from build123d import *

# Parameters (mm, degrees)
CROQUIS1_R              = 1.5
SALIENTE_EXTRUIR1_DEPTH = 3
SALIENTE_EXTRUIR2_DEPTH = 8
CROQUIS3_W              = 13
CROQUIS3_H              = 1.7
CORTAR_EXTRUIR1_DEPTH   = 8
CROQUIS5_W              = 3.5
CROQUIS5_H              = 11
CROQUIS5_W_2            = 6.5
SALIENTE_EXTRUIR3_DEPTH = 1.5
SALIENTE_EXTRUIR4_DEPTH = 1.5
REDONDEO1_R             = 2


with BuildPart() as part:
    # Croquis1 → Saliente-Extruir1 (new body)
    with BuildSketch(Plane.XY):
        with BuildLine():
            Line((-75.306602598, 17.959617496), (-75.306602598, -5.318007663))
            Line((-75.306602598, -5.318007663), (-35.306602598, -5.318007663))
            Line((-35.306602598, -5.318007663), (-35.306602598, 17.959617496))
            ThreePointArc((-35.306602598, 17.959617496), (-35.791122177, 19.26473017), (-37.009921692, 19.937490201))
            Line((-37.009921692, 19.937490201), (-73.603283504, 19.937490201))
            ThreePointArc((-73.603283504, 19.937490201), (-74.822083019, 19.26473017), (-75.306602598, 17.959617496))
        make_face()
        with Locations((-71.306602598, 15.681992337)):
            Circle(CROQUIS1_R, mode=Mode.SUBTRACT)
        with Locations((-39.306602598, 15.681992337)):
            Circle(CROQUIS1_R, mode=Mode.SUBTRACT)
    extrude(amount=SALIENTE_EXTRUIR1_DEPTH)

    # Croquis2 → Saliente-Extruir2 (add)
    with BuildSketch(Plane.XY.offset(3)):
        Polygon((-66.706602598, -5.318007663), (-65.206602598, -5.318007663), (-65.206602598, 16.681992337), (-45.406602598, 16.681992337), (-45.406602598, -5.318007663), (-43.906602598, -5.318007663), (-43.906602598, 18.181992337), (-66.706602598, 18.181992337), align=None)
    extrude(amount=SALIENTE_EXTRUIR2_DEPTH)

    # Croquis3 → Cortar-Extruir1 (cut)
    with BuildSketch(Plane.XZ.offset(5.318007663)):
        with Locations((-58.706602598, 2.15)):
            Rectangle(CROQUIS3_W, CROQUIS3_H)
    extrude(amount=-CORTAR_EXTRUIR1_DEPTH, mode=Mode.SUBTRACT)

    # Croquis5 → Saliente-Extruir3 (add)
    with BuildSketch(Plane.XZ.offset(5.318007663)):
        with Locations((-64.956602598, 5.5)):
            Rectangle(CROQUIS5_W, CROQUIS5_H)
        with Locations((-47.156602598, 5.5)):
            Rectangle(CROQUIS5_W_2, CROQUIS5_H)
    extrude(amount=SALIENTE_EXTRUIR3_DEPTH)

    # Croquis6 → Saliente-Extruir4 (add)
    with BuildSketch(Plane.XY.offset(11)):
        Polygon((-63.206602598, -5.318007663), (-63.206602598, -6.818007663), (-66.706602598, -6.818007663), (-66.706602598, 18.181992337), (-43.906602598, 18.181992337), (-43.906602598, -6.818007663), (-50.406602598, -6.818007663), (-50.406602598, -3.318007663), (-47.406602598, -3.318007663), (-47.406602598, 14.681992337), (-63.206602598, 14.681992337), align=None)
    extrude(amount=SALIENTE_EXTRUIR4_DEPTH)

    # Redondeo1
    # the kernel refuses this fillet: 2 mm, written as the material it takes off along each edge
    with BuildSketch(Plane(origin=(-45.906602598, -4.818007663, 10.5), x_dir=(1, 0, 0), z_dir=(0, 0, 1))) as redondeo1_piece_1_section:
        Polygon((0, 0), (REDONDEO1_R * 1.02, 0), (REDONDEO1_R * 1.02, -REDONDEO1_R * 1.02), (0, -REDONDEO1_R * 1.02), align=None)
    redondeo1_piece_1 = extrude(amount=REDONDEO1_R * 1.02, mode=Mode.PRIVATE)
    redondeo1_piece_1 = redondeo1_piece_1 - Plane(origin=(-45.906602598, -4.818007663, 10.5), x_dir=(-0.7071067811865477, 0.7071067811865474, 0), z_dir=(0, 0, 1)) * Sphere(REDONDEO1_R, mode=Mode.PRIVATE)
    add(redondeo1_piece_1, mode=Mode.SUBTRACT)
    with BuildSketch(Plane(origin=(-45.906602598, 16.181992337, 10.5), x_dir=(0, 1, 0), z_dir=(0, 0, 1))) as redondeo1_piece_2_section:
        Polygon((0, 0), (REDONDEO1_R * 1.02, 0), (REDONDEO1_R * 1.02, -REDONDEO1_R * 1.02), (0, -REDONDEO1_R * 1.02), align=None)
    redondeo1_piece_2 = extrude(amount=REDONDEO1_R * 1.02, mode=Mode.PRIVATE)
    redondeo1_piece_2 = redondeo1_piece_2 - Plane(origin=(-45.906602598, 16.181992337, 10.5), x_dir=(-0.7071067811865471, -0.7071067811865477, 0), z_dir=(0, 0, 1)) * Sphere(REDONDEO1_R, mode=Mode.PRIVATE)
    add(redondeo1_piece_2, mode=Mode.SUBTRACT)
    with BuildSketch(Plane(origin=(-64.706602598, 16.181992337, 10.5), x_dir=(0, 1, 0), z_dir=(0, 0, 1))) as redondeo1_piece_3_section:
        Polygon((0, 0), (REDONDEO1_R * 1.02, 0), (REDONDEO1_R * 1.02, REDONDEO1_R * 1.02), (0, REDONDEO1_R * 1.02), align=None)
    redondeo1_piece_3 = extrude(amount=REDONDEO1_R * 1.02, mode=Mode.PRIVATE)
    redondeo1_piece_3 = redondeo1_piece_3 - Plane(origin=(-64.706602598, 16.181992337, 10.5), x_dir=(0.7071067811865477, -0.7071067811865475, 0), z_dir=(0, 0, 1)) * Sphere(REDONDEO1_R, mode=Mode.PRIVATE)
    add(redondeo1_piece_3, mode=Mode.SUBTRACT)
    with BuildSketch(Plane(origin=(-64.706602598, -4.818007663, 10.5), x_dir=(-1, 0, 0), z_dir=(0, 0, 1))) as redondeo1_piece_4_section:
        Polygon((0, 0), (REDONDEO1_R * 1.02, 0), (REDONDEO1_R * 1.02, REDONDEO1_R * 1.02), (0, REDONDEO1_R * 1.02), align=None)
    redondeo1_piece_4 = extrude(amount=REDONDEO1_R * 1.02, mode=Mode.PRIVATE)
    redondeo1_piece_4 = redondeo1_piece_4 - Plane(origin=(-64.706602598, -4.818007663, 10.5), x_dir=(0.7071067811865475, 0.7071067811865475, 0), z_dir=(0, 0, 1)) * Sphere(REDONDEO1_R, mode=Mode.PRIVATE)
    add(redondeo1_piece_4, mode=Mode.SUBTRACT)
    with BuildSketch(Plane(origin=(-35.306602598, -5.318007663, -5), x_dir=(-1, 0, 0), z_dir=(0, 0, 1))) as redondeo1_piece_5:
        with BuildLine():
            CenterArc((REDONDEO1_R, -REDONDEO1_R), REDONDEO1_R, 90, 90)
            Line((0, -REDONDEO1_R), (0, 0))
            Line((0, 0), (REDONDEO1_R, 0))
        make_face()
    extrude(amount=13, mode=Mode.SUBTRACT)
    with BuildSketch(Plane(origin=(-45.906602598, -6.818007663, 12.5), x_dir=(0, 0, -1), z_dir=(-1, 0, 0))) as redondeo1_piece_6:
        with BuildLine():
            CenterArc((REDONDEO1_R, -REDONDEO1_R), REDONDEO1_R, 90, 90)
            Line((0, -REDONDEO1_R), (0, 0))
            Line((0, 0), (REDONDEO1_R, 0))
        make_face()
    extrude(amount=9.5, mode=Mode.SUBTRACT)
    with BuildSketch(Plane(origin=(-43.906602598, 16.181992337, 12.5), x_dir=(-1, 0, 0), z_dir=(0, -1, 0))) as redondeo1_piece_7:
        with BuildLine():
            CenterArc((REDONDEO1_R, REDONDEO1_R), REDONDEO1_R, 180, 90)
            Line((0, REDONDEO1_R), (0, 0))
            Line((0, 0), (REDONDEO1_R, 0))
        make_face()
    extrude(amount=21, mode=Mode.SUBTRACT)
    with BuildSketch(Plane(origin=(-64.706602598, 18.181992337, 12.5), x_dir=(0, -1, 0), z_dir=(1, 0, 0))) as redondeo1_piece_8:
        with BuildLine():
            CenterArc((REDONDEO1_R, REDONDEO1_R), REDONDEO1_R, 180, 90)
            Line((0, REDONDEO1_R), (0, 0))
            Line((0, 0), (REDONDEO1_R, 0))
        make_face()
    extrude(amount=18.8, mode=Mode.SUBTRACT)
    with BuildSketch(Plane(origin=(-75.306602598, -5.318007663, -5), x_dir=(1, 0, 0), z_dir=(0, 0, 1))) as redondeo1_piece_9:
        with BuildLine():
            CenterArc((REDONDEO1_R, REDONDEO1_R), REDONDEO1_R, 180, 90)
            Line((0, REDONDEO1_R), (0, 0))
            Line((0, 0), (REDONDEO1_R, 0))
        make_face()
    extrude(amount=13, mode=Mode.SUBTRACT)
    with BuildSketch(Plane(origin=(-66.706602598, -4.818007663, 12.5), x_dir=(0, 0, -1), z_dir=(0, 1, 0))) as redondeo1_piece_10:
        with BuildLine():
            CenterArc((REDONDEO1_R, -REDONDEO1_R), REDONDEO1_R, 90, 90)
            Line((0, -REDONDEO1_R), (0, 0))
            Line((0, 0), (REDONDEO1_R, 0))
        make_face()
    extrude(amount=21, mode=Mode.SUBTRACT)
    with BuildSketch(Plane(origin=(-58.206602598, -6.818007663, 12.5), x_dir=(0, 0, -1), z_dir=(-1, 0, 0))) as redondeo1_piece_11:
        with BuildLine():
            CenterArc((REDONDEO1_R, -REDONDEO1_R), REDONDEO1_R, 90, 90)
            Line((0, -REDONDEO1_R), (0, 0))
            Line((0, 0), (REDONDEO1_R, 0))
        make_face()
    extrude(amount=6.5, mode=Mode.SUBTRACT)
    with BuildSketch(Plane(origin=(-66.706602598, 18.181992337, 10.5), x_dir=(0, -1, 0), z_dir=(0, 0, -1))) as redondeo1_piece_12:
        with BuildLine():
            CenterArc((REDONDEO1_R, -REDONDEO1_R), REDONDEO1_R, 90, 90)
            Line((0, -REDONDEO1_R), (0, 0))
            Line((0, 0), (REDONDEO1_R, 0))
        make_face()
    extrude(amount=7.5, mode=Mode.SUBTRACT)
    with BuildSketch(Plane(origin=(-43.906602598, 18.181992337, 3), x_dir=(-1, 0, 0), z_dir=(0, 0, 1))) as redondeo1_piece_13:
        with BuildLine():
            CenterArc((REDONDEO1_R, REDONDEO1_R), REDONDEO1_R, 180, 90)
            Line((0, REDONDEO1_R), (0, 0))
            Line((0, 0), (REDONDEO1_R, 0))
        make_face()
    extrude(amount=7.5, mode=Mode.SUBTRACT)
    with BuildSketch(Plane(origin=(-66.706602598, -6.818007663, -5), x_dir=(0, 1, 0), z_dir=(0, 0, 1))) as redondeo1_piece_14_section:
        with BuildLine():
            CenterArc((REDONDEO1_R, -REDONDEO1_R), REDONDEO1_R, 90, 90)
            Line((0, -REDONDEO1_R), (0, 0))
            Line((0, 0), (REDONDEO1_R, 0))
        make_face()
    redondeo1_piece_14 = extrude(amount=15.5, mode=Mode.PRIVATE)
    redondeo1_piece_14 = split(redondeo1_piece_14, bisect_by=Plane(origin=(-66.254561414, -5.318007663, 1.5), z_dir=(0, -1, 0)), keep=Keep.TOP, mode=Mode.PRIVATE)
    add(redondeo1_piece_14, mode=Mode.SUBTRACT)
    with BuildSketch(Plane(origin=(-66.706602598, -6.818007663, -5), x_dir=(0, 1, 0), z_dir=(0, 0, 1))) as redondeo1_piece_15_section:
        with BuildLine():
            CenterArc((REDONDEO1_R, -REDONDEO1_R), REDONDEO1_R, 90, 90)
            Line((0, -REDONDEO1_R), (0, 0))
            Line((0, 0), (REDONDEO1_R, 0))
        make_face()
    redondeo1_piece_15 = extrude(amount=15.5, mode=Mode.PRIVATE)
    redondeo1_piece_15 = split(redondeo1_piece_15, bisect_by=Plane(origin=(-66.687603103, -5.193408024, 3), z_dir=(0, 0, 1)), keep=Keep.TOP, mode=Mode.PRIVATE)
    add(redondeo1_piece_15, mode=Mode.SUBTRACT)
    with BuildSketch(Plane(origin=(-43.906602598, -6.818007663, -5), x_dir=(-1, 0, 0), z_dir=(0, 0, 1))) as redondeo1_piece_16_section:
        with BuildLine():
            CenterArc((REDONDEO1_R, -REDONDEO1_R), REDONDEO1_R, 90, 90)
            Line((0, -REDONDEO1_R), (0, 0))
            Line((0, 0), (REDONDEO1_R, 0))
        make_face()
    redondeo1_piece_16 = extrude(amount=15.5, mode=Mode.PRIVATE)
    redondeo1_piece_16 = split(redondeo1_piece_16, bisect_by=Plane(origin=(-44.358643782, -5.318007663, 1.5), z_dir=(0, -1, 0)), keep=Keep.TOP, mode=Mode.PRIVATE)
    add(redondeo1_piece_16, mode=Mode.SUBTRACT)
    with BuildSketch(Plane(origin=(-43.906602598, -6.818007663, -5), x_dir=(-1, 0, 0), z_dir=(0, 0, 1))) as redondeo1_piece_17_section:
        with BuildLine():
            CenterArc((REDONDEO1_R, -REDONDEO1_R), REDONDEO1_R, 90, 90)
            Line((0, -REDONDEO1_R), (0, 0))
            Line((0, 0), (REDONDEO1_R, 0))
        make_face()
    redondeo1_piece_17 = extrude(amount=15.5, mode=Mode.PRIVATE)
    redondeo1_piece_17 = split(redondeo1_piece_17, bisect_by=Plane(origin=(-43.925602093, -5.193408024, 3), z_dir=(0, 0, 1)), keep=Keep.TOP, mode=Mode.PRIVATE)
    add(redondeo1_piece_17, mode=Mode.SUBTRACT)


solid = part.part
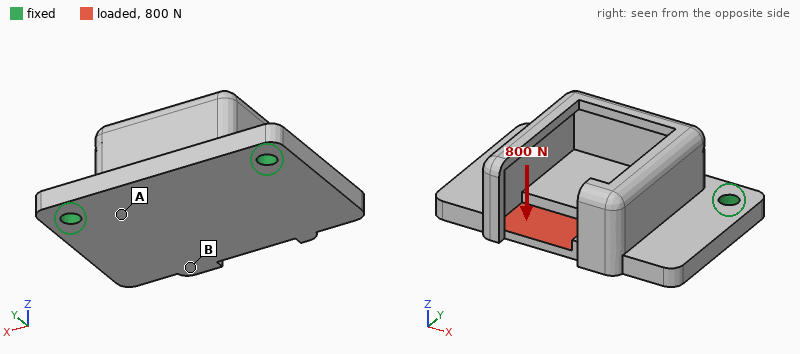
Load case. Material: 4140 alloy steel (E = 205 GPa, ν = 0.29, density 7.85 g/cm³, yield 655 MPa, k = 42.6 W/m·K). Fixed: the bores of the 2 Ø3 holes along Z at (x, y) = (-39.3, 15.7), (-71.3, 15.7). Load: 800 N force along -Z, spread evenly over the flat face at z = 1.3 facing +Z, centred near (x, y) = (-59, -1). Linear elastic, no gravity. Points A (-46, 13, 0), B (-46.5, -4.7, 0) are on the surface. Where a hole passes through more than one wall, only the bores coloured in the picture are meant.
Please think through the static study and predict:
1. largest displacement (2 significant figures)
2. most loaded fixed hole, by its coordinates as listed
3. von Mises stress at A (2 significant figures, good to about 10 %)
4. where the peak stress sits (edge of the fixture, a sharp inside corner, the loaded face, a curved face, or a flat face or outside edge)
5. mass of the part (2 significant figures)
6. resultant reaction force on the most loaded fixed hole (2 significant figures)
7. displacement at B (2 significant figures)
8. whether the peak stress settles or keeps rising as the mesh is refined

0.15 mm
(-71.3, 15.7)
140 MPa
edge of the fixture
32 g
530 N
0.094 mm
keeps rising
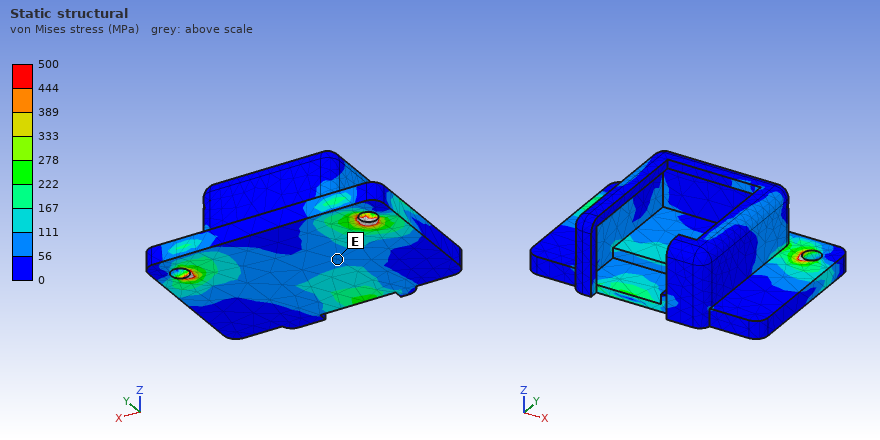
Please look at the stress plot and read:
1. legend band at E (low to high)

56 to 111 MPa
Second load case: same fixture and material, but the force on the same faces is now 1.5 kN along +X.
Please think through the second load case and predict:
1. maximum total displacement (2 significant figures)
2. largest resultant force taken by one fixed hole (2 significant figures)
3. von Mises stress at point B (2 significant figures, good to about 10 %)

9.1 µm
1.1 kN
21 MPa
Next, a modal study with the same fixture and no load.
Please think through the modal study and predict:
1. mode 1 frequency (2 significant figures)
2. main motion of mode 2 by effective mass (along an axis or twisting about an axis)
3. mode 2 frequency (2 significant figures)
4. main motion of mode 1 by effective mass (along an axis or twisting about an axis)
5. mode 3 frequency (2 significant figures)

4300 Hz
twisting about Y
7700 Hz
along Z
10 kHz
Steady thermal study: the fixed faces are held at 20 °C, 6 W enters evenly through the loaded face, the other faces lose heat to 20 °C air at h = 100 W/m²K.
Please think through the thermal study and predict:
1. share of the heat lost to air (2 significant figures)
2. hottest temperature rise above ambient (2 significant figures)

51 %
33 K
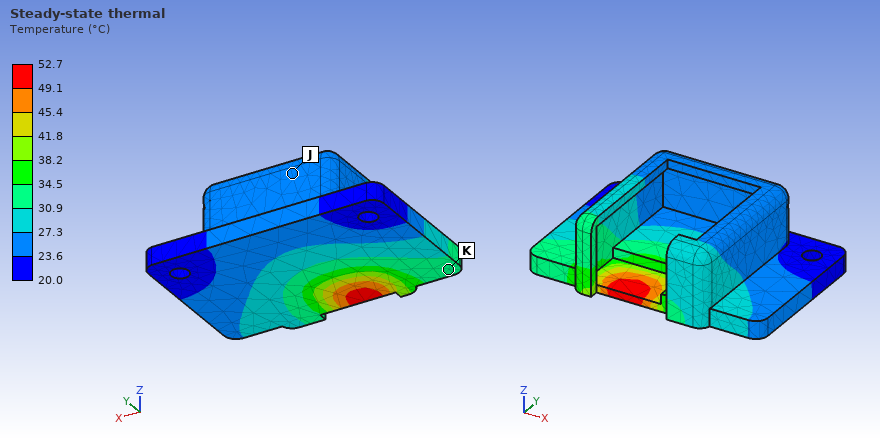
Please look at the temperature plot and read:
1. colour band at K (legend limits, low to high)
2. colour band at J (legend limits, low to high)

30.9 to 34.5 °C
23.6 to 27.3 °C
